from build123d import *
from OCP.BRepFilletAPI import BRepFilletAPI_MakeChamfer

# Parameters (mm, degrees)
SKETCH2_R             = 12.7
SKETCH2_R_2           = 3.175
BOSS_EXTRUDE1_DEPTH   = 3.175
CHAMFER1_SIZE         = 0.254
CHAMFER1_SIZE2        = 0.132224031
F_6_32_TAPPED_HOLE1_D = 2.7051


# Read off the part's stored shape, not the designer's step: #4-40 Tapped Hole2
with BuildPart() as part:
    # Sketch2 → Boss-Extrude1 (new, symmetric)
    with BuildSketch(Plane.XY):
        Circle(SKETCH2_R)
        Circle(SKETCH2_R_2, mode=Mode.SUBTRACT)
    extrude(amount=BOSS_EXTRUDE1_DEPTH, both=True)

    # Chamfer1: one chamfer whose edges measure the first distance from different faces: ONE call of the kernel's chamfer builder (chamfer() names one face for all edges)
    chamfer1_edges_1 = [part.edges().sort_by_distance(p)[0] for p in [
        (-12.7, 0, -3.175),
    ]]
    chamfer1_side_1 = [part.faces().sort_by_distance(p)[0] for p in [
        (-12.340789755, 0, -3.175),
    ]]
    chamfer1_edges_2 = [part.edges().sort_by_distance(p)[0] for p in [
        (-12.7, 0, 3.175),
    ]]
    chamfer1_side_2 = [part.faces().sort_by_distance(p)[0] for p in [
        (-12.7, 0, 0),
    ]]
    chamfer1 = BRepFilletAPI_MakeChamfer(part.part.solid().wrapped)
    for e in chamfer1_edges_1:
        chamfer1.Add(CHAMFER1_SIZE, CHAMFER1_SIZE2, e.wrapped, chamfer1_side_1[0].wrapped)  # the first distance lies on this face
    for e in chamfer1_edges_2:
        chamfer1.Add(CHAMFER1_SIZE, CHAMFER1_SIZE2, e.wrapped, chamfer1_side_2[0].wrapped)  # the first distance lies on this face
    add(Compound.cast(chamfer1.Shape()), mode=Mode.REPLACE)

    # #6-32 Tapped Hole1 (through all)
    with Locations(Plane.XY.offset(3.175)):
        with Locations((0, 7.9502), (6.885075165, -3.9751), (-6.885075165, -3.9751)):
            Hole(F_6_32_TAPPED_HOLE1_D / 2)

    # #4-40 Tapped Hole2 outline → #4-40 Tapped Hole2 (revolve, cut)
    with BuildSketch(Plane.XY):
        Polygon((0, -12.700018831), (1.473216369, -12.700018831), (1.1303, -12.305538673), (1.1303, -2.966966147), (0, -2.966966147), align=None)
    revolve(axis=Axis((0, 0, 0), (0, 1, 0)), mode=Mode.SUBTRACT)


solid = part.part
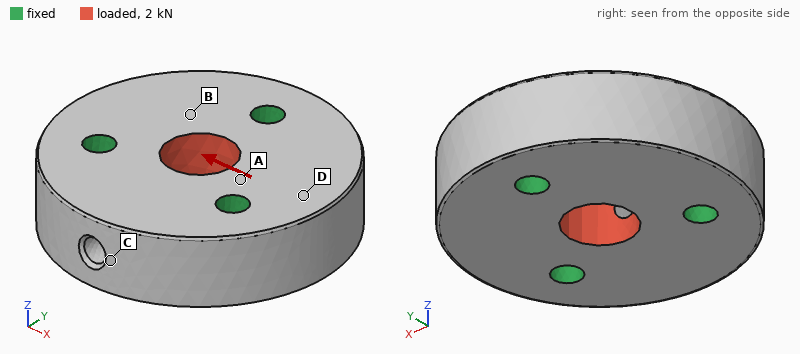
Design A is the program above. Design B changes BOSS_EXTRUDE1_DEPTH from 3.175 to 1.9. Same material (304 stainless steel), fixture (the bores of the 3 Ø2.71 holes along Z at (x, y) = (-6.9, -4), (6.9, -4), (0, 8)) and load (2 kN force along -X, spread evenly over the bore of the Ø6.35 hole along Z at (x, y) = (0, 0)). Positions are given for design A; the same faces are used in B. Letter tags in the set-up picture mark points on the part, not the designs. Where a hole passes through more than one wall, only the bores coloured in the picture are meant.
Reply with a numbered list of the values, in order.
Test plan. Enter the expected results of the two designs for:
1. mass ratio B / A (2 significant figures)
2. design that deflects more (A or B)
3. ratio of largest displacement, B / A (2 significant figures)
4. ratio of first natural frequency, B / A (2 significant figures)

1. 0.59
2. B
3. 1.7
4. 0.75
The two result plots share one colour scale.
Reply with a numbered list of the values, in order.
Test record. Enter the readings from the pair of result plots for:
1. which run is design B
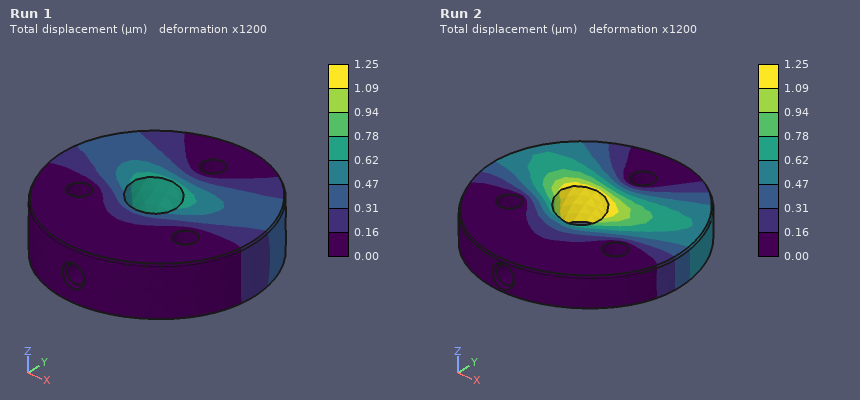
1. Run 2
